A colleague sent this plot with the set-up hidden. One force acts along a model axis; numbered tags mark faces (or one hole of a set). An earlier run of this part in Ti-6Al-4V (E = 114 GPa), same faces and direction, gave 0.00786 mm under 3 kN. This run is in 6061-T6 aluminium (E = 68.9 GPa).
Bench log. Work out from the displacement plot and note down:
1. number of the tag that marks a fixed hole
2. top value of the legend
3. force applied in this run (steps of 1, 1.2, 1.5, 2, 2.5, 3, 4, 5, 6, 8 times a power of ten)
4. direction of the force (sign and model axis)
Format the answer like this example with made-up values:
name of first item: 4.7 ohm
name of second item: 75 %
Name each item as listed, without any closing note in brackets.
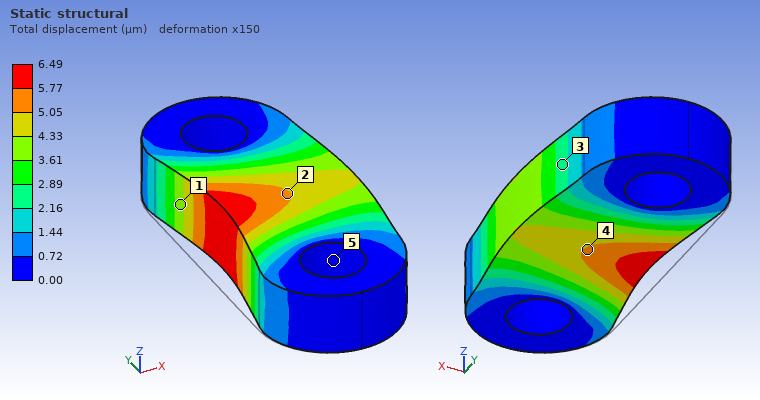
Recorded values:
number of the tag that marks a fixed hole: 5
top value of the legend: 6.49 µm
force applied in this run: 1.5 kN
direction of the force: +X
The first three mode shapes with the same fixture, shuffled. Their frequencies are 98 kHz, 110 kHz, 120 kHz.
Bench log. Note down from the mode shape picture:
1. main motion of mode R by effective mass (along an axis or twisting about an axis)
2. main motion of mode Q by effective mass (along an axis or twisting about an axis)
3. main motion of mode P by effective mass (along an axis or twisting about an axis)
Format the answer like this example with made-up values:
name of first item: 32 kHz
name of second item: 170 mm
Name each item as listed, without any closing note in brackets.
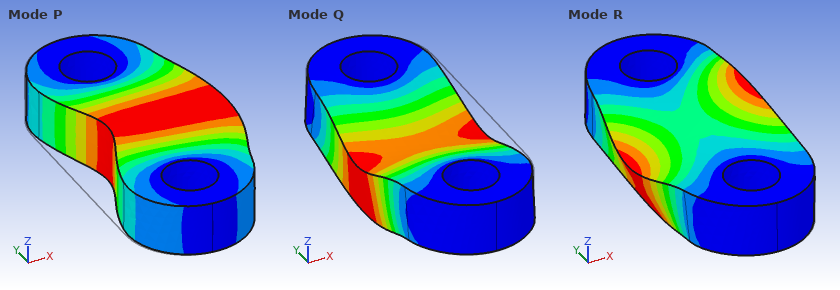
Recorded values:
main motion of mode R by effective mass: twisting about Y
main motion of mode Q by effective mass: along Z
main motion of mode P by effective mass: along X
